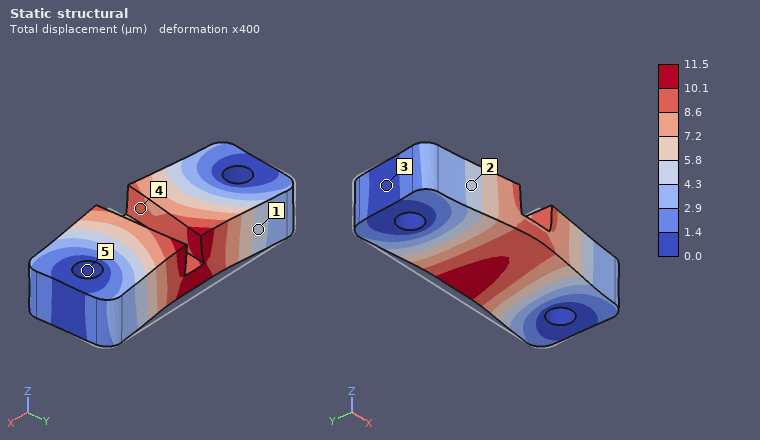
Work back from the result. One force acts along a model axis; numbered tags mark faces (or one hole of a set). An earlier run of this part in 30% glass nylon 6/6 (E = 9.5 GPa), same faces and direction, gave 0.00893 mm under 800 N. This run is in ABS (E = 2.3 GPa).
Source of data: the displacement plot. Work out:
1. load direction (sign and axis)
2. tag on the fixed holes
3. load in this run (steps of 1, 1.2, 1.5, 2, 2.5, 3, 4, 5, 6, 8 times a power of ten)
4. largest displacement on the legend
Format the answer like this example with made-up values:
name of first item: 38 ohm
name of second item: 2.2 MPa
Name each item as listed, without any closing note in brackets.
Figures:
load direction: -Y
tag on the fixed holes: 5
load in this run: 250 N
largest displacement on the legend: 11.5 µm
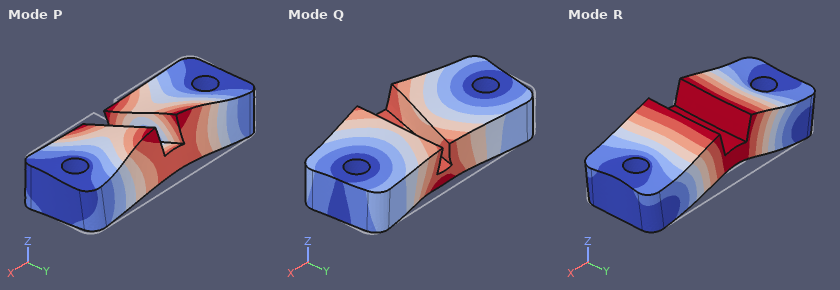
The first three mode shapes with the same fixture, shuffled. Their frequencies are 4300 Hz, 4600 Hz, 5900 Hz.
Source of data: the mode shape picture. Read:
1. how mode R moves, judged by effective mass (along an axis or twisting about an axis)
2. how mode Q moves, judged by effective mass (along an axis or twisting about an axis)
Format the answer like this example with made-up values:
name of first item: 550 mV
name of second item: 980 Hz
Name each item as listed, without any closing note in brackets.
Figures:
how mode R moves, judged by effective mass: along Z
how mode Q moves, judged by effective mass: along Y
